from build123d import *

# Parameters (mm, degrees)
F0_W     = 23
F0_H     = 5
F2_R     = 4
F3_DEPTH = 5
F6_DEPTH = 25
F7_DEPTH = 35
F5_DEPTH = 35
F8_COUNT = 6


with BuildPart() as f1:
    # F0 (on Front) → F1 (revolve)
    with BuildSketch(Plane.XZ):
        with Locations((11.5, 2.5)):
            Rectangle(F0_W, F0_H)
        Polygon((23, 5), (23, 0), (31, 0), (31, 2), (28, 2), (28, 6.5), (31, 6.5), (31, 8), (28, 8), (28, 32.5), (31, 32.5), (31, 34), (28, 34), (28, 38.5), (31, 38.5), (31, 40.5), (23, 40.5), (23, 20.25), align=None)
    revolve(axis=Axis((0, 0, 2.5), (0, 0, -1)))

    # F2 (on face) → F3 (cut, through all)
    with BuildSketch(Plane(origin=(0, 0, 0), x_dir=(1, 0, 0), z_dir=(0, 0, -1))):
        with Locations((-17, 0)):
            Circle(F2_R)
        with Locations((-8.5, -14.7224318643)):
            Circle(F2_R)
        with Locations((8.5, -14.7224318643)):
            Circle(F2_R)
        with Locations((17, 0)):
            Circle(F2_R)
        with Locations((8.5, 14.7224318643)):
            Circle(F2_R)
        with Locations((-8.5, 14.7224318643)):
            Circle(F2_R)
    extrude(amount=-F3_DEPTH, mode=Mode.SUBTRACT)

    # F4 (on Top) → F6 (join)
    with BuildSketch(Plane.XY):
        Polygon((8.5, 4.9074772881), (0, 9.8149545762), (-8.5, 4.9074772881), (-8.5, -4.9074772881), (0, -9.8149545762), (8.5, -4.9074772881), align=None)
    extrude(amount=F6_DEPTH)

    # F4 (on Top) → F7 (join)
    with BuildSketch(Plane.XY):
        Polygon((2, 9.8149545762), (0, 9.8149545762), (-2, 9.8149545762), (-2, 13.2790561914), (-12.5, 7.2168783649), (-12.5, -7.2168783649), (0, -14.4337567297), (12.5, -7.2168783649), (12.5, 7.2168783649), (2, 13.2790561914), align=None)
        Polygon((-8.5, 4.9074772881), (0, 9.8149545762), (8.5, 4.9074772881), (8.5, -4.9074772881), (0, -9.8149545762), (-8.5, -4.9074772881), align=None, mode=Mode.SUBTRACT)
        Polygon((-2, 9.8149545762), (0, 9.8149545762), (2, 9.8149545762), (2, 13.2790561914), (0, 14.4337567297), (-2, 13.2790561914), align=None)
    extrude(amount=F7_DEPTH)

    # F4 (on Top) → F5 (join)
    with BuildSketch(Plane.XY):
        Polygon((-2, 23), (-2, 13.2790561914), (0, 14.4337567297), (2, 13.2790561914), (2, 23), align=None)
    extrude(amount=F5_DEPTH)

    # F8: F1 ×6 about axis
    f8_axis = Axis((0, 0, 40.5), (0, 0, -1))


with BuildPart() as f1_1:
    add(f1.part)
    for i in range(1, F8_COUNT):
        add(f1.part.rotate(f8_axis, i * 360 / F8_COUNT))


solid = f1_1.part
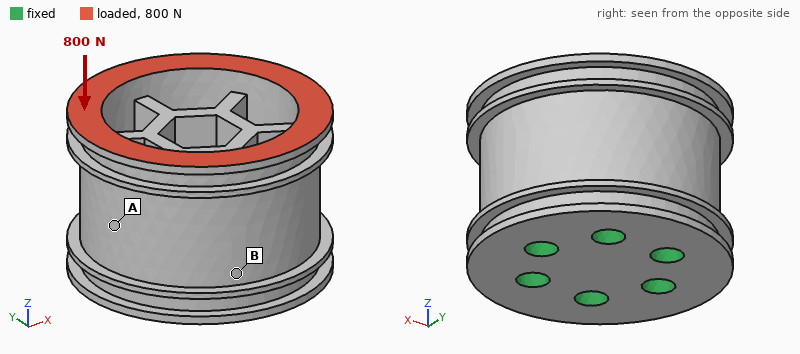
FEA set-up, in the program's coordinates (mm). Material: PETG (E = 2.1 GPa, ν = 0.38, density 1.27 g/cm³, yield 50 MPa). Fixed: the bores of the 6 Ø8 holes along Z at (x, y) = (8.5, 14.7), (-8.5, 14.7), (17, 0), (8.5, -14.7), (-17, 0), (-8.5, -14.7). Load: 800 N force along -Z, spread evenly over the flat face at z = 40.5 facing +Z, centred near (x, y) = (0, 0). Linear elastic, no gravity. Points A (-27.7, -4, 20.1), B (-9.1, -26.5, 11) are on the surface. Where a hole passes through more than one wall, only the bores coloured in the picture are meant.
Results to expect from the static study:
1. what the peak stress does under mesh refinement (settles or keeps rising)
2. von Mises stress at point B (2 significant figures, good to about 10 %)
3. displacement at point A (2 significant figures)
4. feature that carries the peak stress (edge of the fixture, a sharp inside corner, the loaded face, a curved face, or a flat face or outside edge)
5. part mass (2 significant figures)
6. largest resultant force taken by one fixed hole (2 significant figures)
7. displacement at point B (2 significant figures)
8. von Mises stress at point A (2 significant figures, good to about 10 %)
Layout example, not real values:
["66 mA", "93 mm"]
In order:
["keeps rising", "0.48 MPa", "15 µm", "edge of the fixture", "81 g", "130 N", "12 µm", "0.80 MPa"]
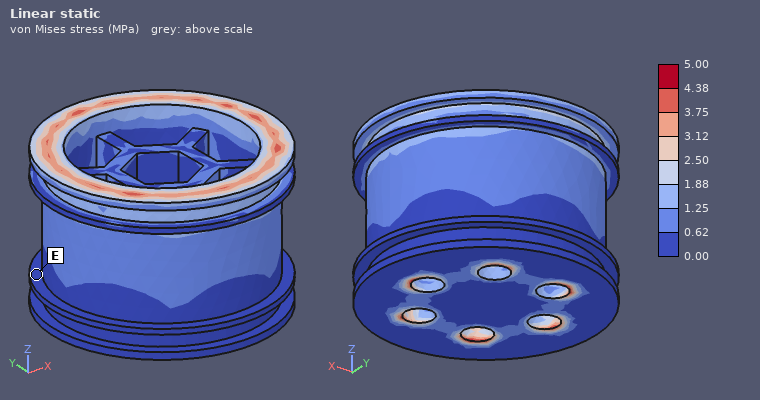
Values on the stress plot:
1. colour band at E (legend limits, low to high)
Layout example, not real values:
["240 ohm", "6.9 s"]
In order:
["0.00 to 0.62 MPa"]
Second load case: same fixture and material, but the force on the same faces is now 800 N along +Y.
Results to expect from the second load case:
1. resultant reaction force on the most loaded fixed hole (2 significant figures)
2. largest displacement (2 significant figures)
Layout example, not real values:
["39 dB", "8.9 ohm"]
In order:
["460 N", "0.21 mm"]
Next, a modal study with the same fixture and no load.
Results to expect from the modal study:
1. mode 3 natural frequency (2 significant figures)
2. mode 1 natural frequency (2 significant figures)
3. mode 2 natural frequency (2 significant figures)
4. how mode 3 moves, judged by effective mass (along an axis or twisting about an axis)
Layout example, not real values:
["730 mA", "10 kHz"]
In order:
["4000 Hz", "2500 Hz", "2500 Hz", "twisting about Z"]
